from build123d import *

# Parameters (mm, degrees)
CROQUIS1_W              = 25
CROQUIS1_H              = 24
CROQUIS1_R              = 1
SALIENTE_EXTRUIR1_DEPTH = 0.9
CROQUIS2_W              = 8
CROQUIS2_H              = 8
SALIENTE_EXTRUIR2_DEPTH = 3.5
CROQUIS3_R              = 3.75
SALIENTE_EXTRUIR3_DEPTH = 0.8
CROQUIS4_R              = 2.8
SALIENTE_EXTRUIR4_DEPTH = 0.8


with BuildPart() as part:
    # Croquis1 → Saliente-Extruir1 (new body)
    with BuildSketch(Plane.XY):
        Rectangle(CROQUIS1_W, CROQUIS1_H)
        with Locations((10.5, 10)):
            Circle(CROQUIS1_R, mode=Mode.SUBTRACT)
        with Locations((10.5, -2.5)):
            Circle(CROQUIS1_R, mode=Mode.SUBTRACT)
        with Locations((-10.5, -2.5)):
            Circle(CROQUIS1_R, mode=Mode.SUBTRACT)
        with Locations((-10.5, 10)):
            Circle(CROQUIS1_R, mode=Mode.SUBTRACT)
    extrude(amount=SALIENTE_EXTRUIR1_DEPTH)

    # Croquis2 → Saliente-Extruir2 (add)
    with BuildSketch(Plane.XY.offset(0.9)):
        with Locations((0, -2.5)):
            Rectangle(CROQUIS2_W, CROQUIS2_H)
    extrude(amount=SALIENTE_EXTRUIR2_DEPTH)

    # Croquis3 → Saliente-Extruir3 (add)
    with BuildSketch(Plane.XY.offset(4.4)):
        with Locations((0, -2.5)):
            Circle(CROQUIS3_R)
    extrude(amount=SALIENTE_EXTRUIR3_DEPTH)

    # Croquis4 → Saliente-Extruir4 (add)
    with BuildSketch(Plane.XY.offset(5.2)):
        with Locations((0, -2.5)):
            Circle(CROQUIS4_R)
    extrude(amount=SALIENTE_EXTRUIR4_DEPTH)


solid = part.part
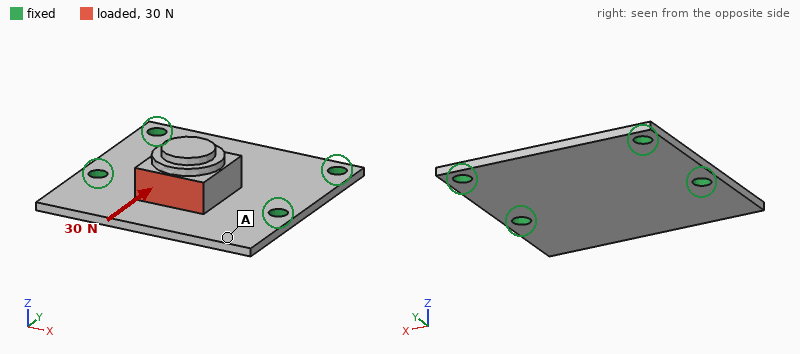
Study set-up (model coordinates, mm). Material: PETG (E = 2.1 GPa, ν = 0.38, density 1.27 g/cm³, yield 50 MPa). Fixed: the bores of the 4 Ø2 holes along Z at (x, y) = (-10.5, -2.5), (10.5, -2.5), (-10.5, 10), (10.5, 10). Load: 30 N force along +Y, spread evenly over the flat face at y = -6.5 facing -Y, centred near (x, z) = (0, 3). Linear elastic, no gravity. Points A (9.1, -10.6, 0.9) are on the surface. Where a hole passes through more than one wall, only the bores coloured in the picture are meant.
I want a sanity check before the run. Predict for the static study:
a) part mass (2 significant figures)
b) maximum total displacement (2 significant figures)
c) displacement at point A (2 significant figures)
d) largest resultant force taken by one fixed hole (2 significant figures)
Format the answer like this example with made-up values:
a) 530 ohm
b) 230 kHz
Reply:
a) 1.0 g
b) 0.32 mm
c) 0.17 mm
d) 9.5 N
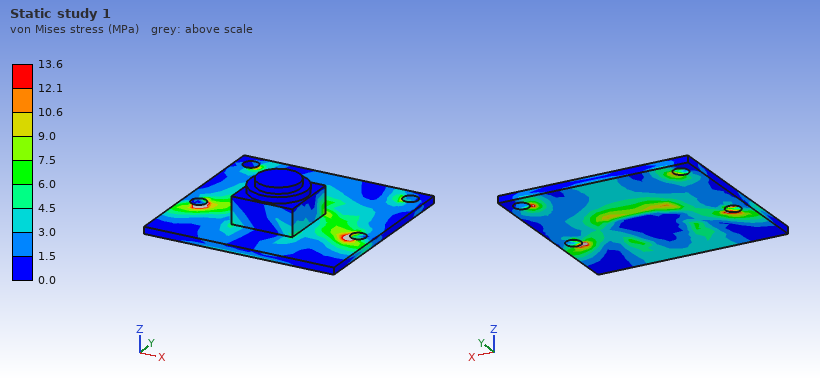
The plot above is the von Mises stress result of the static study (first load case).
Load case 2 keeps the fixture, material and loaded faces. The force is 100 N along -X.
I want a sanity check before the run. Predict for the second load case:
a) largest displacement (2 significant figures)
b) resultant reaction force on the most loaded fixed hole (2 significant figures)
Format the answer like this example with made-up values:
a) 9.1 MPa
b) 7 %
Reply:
a) 0.21 mm
b) 48 N
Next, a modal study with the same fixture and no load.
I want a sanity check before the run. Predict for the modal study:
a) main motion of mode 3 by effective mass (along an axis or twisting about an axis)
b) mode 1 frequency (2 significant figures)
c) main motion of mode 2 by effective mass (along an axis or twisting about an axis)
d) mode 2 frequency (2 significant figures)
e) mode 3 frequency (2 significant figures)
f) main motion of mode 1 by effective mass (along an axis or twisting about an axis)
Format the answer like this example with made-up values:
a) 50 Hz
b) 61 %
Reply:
a) twisting about Y
b) 1700 Hz
c) along Z
d) 2500 Hz
e) 3400 Hz
f) along Z
